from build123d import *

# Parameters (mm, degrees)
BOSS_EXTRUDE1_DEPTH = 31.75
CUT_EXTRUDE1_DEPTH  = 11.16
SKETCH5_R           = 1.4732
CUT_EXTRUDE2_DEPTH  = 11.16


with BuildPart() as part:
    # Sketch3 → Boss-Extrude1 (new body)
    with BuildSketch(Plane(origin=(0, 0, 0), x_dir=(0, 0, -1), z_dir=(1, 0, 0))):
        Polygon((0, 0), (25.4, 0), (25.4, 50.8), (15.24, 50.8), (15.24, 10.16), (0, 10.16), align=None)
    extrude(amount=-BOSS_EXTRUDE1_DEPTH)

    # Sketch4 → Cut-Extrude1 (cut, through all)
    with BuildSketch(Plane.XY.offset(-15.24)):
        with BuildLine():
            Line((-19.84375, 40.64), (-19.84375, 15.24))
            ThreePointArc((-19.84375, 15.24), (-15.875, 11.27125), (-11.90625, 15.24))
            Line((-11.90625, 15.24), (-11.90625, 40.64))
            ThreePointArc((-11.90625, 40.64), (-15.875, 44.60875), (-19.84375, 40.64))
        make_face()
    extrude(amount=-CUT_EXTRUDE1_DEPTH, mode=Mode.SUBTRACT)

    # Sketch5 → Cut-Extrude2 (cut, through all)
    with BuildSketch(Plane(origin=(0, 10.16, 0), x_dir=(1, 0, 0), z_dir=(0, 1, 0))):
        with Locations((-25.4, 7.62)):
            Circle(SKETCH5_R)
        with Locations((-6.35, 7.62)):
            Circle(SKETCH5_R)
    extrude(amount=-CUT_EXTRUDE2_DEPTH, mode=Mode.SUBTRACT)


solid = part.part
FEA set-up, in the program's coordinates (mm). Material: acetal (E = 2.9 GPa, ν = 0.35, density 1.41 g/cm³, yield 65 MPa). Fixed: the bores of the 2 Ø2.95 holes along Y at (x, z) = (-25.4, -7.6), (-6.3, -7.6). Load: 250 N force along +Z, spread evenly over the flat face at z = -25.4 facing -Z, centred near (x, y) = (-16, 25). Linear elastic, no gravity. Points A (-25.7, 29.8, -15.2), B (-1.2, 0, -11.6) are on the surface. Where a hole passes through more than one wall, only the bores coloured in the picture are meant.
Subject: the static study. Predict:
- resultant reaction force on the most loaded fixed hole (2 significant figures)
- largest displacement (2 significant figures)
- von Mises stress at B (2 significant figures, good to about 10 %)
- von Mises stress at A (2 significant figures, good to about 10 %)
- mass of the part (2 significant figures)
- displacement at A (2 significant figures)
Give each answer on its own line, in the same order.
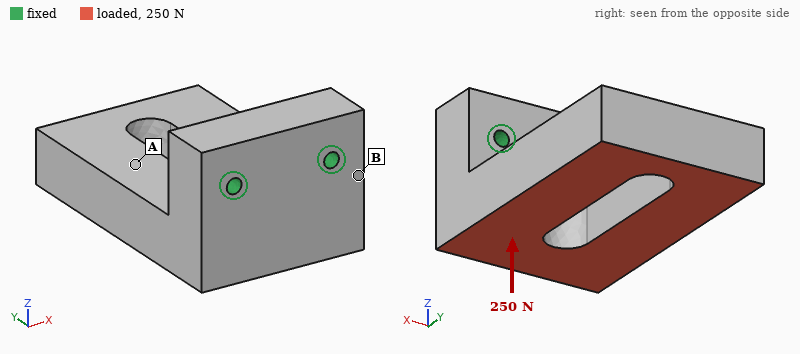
130 N
0.75 mm
7.3 MPa
2.8 MPa
26 g
0.34 mm
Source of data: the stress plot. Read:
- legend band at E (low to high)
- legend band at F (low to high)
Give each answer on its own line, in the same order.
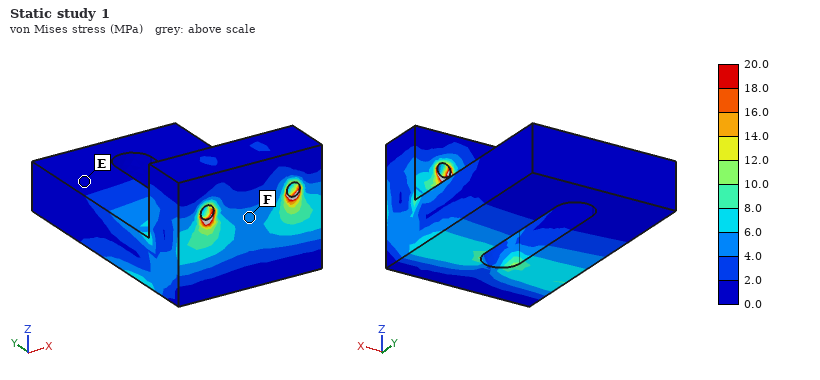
0.0 to 2.0 MPa
4.0 to 6.0 MPa
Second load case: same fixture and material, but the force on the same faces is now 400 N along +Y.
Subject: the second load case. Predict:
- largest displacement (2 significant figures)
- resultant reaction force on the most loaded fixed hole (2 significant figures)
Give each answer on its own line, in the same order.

0.61 mm
200 N
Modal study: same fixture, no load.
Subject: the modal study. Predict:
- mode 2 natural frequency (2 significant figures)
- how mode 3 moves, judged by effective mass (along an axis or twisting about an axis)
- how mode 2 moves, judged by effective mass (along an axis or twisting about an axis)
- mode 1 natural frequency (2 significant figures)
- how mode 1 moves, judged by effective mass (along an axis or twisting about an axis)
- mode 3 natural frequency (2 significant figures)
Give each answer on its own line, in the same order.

1300 Hz
twisting about Y
along X
790 Hz
along Z
2300 Hz
